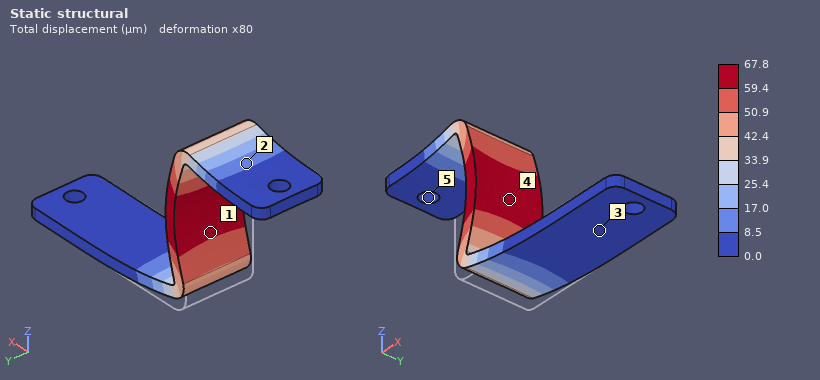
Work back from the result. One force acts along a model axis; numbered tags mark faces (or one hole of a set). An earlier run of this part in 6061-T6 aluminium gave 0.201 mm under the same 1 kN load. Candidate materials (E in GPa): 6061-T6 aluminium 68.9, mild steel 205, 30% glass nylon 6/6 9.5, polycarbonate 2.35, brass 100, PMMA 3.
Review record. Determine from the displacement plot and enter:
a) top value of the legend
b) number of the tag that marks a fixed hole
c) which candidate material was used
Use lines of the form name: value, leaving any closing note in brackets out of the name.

top value of the legend: 67.8 µm
number of the tag that marks a fixed hole: 5
which candidate material was used: mild steel
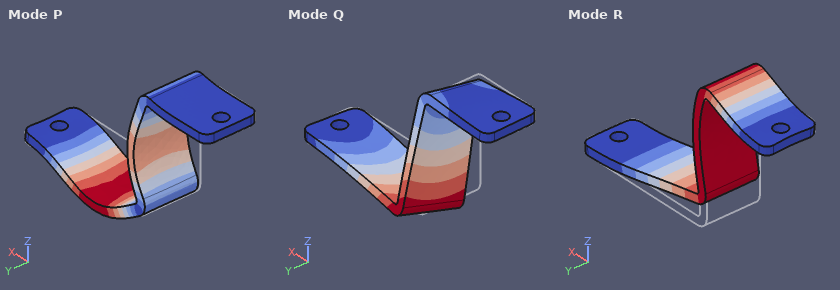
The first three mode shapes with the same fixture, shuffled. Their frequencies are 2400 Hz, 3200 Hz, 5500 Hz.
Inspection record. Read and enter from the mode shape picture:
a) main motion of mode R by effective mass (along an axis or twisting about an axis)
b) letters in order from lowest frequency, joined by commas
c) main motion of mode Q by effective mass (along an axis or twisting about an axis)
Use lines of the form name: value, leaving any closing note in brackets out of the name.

main motion of mode R by effective mass: along Z
letters in order from lowest frequency, joined by commas: R, Q, P
main motion of mode Q by effective mass: along Y
